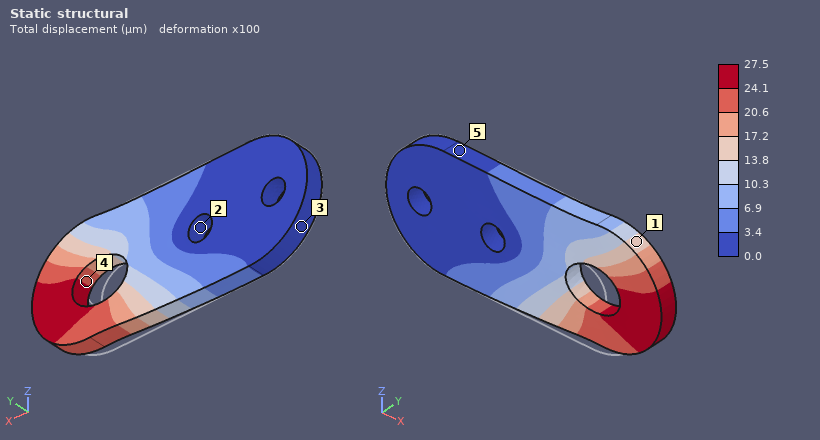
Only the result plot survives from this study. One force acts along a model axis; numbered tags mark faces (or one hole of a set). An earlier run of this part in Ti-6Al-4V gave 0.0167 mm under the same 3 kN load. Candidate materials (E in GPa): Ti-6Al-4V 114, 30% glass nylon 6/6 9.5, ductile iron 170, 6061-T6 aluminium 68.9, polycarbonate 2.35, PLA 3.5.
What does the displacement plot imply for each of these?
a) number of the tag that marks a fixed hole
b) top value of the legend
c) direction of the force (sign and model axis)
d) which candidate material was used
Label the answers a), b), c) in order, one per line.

a) 2
b) 27.5 µm
c) +X
d) 6061-T6 aluminium
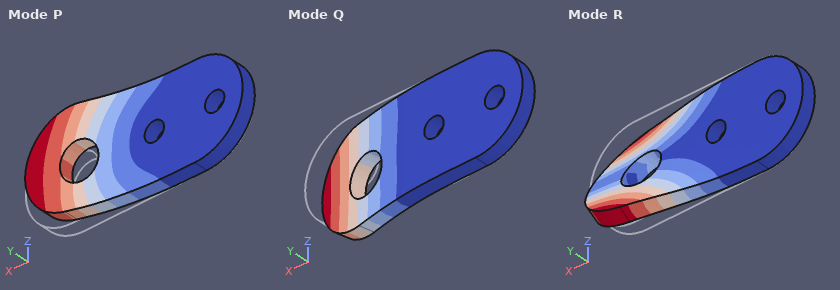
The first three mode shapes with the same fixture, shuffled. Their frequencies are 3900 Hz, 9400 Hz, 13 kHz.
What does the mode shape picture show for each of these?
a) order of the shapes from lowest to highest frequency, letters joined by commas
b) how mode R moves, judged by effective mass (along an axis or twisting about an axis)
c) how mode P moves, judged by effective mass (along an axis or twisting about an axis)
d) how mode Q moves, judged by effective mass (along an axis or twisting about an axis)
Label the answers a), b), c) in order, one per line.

a) Q, R, P
b) twisting about X
c) along Z
d) along Y
